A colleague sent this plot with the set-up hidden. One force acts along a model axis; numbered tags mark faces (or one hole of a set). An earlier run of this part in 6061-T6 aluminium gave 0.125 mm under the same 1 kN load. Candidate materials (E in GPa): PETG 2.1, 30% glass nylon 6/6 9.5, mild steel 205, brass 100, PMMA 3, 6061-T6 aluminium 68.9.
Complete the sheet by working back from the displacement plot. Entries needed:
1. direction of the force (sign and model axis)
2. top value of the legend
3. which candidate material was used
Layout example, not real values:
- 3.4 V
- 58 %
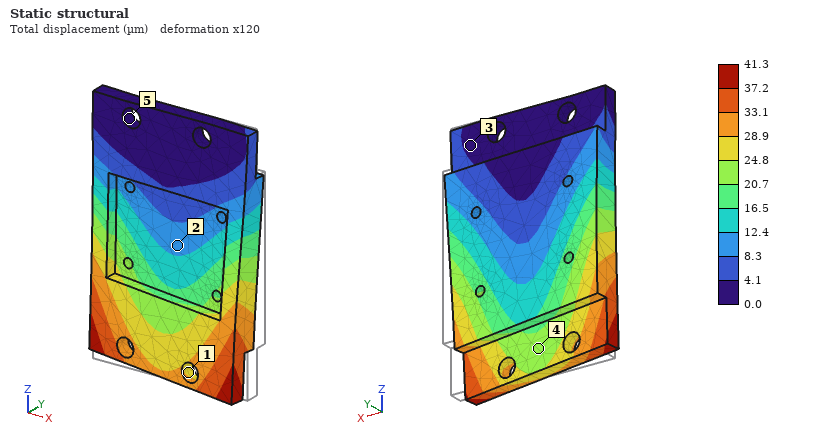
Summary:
- -X
- 41.3 µm
- mild steel
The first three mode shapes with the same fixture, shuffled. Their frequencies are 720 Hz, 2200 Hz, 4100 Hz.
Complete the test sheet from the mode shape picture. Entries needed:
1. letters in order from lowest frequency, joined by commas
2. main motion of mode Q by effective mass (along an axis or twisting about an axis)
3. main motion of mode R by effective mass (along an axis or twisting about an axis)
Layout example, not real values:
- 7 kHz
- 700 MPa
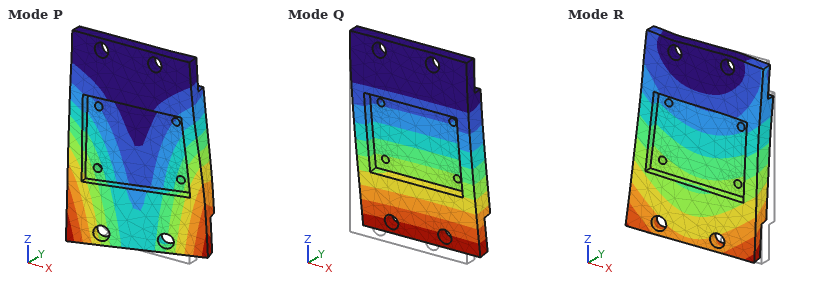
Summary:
- Q, P, R
- along Y
- along X
